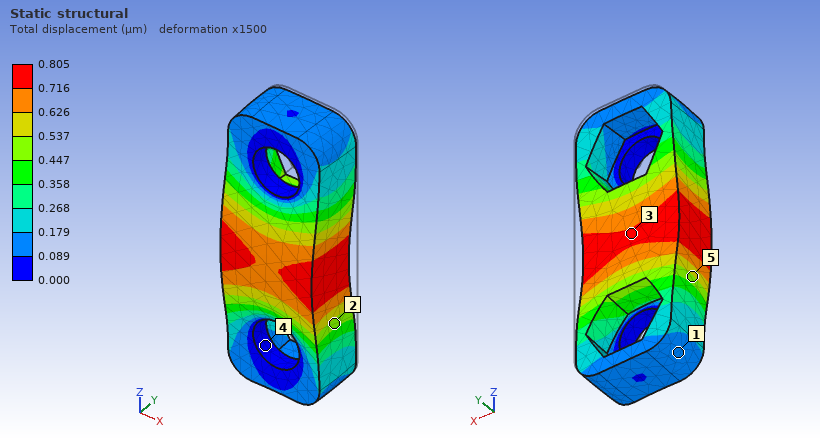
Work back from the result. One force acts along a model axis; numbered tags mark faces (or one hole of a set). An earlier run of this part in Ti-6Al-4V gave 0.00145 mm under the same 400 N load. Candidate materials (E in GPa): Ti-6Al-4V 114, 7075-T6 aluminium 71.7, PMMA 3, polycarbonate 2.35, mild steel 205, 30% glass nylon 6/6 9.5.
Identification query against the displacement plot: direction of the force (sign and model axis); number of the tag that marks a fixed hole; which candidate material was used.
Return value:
-Y
4
mild steel
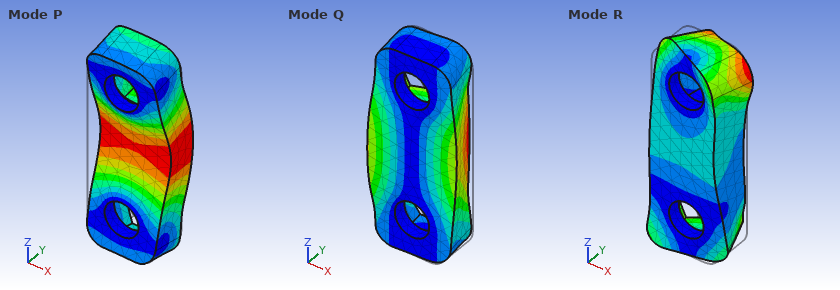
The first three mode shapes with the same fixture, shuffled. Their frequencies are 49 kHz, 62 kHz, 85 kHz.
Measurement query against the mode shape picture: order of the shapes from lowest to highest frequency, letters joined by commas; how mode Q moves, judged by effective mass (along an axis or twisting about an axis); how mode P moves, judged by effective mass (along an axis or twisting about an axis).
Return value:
Q, P, R
along X
along Y
